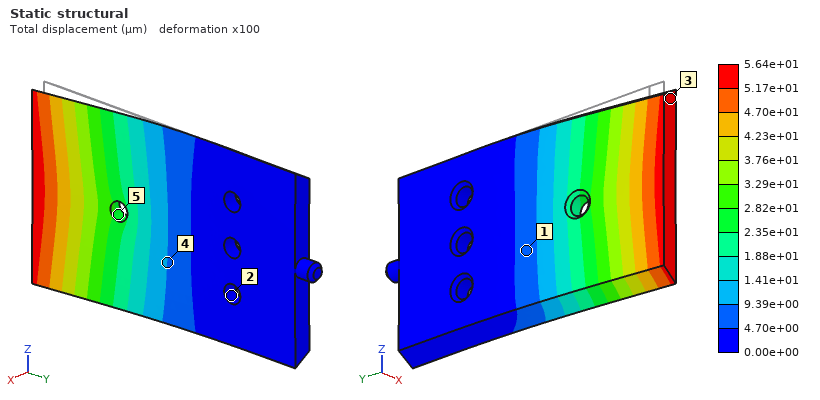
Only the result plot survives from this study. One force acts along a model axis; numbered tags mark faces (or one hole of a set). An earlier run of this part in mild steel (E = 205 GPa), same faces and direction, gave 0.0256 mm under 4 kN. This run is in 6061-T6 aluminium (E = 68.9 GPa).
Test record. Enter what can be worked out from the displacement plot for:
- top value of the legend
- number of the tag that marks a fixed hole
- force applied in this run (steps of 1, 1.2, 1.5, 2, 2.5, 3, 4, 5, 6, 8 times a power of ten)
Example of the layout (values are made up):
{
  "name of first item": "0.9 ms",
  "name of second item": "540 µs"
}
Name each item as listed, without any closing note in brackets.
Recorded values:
{
  "top value of the legend": "5.64e+01 µm",
  "number of the tag that marks a fixed hole": "2",
  "force applied in this run": "3 kN"
}
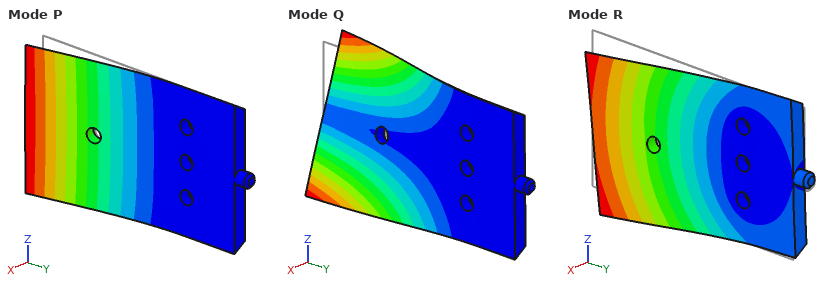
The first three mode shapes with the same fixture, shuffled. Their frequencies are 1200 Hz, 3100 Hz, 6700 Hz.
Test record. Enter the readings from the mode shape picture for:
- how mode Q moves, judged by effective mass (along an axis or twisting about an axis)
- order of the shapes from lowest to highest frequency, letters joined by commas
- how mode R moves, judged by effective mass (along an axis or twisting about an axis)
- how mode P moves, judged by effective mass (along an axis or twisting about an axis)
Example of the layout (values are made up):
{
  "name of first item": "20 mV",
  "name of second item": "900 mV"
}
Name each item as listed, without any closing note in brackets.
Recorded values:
{
  "how mode Q moves, judged by effective mass": "twisting about Y",
  "order of the shapes from lowest to highest frequency, letters joined by commas": "P, Q, R",
  "how mode R moves, judged by effective mass": "along Z",
  "how mode P moves, judged by effective mass": "along X"
}
